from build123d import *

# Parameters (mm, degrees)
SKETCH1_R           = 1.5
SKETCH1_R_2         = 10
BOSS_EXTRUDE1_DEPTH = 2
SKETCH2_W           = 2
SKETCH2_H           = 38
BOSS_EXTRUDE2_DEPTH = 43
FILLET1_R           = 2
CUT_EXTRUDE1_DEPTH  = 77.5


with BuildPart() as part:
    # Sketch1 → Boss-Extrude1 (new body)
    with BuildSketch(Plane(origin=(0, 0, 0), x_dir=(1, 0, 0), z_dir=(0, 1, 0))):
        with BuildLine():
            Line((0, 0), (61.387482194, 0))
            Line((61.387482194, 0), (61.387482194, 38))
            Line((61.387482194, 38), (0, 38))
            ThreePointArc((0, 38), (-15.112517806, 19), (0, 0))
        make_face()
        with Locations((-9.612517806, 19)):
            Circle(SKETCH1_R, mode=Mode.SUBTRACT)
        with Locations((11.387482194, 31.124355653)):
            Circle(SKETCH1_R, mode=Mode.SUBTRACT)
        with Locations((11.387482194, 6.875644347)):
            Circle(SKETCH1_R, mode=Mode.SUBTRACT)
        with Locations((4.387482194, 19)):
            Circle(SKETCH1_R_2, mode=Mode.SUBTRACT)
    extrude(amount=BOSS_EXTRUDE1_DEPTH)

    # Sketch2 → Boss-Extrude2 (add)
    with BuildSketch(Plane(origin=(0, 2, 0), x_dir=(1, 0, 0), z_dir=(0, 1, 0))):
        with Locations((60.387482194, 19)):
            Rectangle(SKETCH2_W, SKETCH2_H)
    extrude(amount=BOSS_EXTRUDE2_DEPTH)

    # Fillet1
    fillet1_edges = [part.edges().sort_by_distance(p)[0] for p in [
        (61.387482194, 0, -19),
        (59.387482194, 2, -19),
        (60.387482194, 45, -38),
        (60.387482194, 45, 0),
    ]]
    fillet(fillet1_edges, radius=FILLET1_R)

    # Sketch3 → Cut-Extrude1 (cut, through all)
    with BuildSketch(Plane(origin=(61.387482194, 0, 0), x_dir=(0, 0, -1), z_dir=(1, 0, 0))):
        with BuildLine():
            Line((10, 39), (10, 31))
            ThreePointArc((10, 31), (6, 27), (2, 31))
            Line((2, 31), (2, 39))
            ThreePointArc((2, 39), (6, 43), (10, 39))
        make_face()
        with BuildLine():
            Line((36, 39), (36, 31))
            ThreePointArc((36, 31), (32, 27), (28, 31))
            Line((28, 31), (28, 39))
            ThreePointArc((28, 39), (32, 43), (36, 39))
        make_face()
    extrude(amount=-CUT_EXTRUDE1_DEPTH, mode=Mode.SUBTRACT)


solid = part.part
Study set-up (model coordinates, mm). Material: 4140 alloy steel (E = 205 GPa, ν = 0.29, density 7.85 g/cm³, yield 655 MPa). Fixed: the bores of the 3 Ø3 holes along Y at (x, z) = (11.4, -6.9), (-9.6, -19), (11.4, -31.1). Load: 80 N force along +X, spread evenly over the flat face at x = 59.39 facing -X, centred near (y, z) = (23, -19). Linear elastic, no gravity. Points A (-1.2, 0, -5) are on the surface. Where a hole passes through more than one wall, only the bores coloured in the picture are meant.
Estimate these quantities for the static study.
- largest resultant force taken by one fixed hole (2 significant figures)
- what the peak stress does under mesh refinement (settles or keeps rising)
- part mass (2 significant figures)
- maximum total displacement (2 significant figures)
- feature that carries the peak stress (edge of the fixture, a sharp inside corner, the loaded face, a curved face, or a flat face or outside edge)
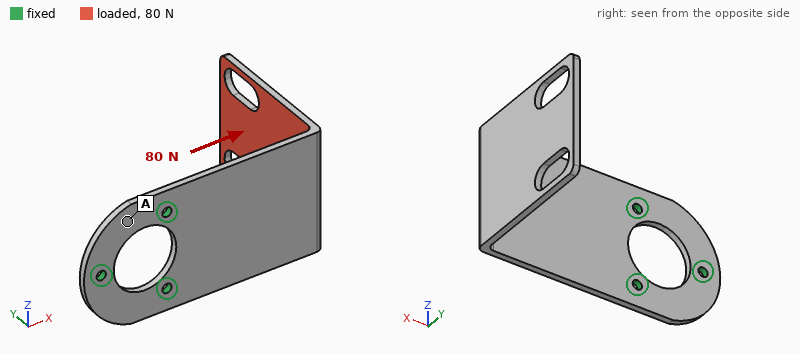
40 N
keeps rising
60 g
0.95 mm
edge of the fixture
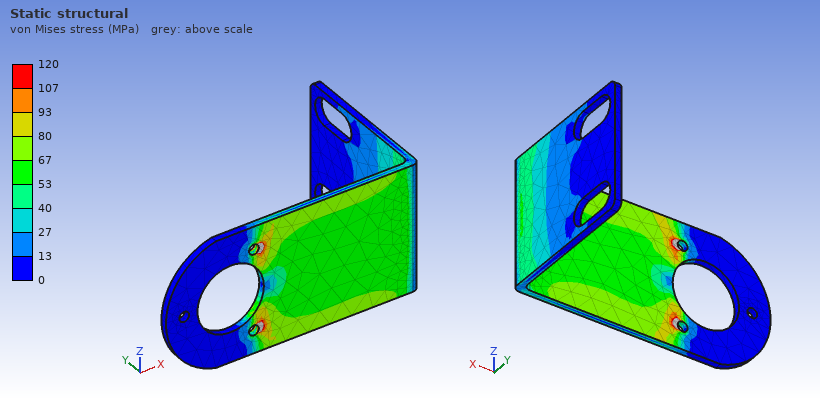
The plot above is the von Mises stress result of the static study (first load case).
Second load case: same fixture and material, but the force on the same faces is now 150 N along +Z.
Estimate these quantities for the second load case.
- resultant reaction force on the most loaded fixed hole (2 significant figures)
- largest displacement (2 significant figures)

290 N
0.69 mm
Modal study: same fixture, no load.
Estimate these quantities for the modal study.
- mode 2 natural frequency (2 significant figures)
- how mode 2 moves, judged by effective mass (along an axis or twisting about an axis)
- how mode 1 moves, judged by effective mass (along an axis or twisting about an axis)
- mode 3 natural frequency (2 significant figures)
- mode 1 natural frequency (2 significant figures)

590 Hz
along Z
along Y
830 Hz
270 Hz
